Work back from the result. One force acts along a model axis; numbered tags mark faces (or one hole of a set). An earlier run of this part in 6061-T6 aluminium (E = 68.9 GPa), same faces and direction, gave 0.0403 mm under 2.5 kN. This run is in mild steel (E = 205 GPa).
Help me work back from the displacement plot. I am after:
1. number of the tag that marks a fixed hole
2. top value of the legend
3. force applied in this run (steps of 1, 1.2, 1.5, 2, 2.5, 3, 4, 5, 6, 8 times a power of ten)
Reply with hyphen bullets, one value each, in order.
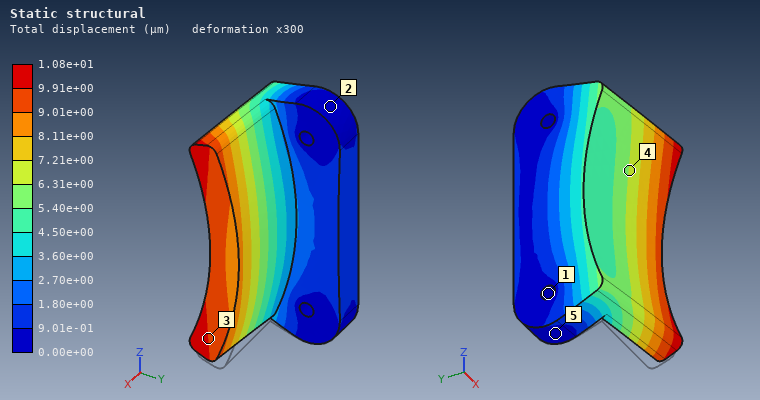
- 1
- 1.08e+01 µm
- 2 kN
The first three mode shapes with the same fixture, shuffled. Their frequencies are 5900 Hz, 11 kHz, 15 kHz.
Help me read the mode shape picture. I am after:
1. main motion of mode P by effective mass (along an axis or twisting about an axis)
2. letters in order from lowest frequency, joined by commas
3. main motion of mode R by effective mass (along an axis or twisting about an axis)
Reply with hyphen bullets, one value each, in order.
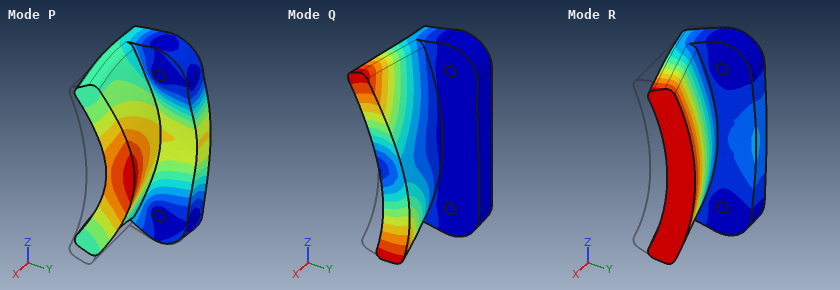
- along X
- R, Q, P
- along Y
